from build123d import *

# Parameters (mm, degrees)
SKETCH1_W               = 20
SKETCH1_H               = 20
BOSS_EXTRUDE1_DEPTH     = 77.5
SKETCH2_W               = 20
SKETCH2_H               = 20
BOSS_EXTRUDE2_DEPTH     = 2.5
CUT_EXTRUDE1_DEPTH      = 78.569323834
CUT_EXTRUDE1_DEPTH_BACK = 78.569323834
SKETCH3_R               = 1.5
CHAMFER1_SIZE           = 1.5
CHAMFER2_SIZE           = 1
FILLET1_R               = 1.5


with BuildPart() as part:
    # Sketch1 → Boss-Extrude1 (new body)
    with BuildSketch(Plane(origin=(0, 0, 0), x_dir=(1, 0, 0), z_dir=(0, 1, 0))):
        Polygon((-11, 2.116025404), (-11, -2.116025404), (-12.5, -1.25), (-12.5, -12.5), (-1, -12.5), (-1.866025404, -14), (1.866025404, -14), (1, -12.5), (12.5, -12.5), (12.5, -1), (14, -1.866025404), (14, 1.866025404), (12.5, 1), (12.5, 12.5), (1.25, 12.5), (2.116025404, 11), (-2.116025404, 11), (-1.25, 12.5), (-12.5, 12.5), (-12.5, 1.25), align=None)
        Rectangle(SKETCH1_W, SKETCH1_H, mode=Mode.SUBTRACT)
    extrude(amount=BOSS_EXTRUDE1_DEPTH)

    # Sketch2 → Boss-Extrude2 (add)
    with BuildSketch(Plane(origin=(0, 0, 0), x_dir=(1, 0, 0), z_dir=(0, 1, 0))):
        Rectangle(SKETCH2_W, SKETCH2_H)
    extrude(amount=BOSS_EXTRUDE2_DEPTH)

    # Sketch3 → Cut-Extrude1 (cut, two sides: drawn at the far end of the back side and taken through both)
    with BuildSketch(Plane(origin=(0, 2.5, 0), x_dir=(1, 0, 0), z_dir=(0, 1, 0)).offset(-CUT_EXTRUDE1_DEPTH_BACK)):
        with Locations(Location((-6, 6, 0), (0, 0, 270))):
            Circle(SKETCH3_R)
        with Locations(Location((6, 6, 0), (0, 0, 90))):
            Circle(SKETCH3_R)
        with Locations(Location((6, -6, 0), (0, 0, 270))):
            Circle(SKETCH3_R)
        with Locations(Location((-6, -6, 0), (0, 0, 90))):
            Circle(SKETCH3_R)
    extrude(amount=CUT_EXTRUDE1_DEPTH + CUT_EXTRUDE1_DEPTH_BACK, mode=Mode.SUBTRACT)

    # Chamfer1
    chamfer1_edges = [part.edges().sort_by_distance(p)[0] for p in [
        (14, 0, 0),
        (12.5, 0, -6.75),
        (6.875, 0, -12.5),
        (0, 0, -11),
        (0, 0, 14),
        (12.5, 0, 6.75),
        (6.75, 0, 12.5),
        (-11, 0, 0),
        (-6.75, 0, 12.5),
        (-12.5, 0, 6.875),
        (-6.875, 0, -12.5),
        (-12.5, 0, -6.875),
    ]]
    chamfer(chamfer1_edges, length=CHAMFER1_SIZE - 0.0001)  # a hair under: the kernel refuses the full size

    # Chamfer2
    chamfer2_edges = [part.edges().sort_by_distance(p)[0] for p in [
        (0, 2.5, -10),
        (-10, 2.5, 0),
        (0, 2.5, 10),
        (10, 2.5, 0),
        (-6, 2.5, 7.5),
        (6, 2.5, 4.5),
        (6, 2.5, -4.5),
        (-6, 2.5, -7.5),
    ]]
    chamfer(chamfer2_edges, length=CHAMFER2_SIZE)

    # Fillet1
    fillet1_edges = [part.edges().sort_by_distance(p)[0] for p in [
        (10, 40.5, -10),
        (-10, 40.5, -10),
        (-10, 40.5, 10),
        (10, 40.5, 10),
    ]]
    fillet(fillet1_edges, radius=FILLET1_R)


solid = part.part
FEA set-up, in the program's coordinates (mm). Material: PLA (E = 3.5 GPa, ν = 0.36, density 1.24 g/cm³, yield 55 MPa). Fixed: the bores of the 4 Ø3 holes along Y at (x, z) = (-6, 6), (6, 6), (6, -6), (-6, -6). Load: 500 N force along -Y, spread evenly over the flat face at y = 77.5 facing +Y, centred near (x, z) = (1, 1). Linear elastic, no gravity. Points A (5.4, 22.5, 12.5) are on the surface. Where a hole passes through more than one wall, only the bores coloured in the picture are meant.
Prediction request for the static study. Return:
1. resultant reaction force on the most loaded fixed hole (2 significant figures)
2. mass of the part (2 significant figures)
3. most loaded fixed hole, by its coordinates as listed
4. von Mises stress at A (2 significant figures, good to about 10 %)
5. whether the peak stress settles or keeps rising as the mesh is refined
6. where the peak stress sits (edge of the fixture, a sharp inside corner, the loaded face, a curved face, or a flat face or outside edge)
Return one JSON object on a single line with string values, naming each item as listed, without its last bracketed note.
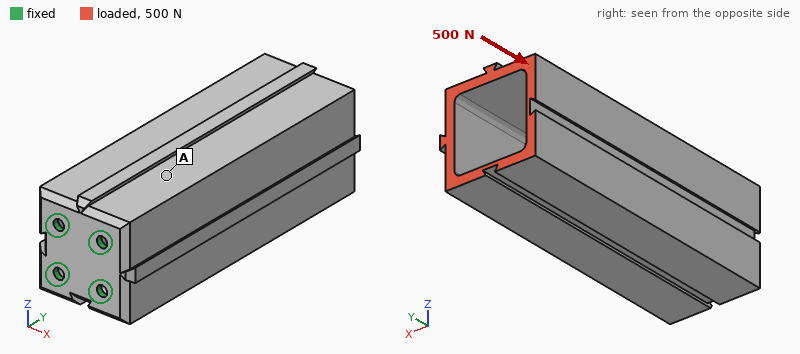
{"resultant reaction force on the most loaded fixed hole": "150 N", "mass of the part": "23 g", "most loaded fixed hole, by its coordinates as listed": "(6, 6)", "von Mises stress at A": "2.4 MPa", "whether the peak stress settles or keeps rising as the mesh is refined": "keeps rising", "where the peak stress sits": "edge of the fixture"}
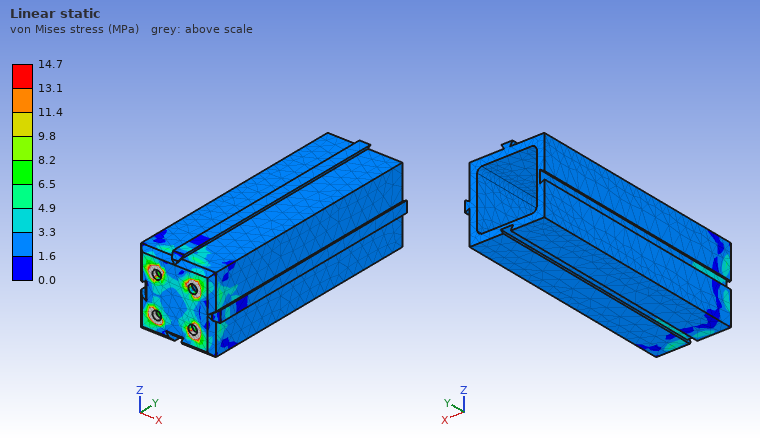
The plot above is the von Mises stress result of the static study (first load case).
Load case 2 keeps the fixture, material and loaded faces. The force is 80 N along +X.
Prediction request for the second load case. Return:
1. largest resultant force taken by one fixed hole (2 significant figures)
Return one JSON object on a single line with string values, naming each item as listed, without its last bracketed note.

{"largest resultant force taken by one fixed hole": "220 N"}
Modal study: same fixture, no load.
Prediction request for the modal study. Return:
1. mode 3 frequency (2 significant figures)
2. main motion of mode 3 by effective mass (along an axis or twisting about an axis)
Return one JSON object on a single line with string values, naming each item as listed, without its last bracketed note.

{"mode 3 frequency": "2500 Hz", "main motion of mode 3 by effective mass": "twisting about Y"}
